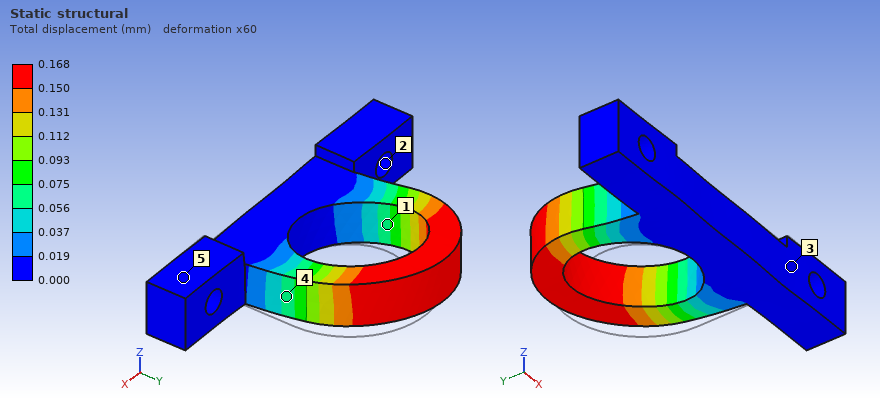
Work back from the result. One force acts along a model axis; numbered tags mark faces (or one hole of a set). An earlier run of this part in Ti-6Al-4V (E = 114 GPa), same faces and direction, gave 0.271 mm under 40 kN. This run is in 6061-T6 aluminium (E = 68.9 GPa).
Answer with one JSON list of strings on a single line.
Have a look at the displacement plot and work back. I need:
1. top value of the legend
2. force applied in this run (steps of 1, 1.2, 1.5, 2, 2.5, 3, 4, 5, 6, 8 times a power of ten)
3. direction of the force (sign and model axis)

["0.168 mm", "15 kN", "-X"]
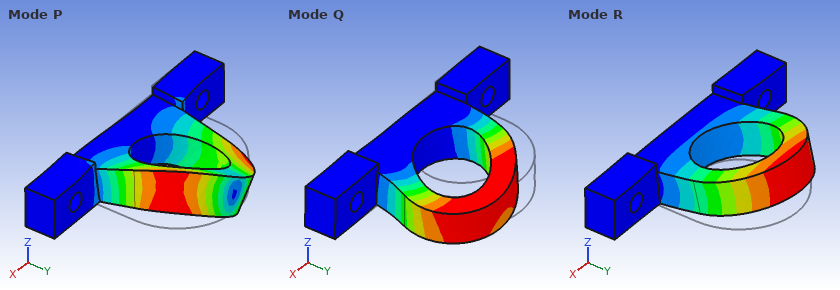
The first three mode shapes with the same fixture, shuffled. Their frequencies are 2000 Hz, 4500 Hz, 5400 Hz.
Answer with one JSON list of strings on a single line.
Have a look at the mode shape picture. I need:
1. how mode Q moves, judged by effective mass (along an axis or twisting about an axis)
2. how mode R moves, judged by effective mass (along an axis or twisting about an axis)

["along X", "along Z"]
